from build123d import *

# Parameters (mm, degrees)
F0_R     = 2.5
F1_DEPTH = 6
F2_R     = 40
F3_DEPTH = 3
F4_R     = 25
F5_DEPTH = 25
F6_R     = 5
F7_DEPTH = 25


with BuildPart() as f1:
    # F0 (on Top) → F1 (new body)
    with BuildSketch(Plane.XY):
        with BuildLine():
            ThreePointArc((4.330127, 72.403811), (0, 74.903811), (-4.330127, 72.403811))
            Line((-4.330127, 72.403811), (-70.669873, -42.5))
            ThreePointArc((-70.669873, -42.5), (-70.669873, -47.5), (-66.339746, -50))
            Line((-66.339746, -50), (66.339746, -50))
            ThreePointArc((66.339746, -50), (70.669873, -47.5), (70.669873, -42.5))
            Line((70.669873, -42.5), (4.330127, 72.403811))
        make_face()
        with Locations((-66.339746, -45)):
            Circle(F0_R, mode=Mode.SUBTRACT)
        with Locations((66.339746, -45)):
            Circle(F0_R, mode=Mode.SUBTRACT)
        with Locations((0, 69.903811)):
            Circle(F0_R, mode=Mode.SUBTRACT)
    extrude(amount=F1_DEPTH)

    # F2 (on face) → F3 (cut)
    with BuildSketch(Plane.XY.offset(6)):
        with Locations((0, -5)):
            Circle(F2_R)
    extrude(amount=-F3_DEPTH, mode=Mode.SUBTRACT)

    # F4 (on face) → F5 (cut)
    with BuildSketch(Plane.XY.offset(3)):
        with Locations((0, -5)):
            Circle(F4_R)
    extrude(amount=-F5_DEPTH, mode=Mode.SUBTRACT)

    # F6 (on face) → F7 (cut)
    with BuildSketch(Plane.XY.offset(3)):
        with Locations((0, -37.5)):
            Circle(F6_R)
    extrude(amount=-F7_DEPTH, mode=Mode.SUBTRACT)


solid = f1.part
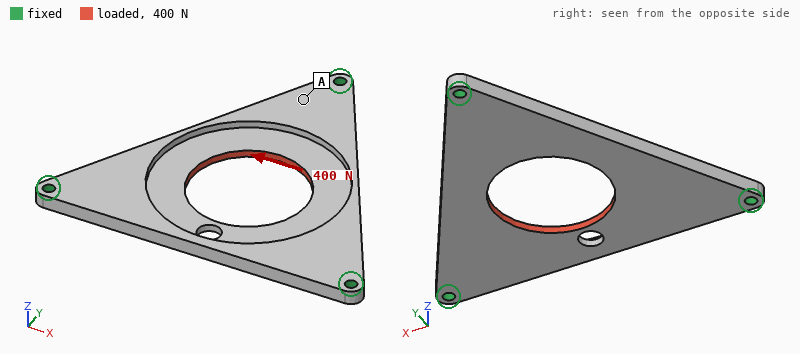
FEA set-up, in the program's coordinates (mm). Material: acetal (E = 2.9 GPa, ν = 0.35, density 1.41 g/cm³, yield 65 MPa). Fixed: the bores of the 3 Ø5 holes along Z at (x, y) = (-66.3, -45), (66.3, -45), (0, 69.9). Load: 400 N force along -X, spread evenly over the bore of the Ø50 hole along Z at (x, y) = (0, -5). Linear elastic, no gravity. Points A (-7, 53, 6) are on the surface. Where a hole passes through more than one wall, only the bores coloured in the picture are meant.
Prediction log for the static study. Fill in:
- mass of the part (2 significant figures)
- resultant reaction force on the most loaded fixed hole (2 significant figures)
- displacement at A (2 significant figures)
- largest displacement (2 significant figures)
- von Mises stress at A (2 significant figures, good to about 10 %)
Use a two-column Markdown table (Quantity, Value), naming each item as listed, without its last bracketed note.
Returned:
| Quantity | Value |
|---|---|
| mass of the part | 52 g |
| resultant reaction force on the most loaded fixed hole | 180 N |
| displacement at A | 0.052 mm |
| largest displacement | 0.14 mm |
| von Mises stress at A | 0.98 MPa |
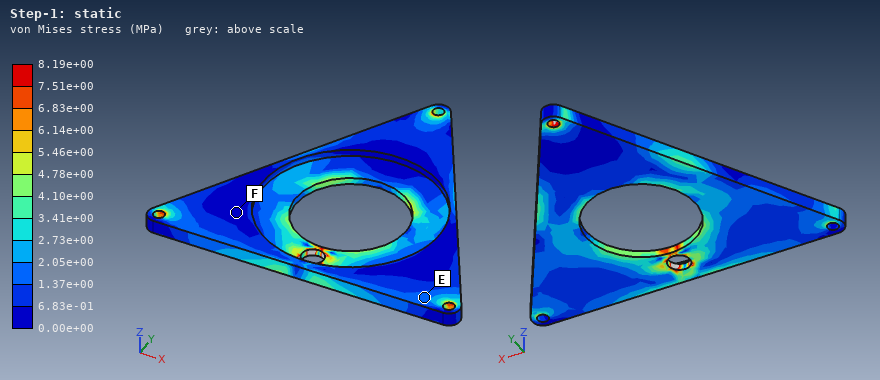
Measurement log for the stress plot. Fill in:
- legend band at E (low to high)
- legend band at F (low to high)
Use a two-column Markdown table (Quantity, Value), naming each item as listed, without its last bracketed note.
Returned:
| Quantity | Value |
|---|---|
| legend band at E | 1.37e+00 to 2.05e+00 MPa |
| legend band at F | 0.00e+00 to 6.83e-01 MPa |
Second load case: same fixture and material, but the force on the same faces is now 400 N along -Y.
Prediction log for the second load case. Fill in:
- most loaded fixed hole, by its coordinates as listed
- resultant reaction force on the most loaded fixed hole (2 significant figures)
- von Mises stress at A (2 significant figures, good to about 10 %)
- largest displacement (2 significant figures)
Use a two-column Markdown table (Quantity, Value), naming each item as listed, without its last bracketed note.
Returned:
| Quantity | Value |
|---|---|
| most loaded fixed hole, by its coordinates as listed | (0, 69.9) |
| resultant reaction force on the most loaded fixed hole | 200 N |
| von Mises stress at A | 1.1 MPa |
| largest displacement | 0.15 mm |
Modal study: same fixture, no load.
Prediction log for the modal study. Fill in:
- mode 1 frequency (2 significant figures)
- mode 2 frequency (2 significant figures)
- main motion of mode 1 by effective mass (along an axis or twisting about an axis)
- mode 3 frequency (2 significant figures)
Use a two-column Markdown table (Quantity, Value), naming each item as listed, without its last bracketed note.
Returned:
| Quantity | Value |
|---|---|
| mode 1 frequency | 410 Hz |
| mode 2 frequency | 580 Hz |
| main motion of mode 1 by effective mass | along Z |
| mode 3 frequency | 590 Hz |
